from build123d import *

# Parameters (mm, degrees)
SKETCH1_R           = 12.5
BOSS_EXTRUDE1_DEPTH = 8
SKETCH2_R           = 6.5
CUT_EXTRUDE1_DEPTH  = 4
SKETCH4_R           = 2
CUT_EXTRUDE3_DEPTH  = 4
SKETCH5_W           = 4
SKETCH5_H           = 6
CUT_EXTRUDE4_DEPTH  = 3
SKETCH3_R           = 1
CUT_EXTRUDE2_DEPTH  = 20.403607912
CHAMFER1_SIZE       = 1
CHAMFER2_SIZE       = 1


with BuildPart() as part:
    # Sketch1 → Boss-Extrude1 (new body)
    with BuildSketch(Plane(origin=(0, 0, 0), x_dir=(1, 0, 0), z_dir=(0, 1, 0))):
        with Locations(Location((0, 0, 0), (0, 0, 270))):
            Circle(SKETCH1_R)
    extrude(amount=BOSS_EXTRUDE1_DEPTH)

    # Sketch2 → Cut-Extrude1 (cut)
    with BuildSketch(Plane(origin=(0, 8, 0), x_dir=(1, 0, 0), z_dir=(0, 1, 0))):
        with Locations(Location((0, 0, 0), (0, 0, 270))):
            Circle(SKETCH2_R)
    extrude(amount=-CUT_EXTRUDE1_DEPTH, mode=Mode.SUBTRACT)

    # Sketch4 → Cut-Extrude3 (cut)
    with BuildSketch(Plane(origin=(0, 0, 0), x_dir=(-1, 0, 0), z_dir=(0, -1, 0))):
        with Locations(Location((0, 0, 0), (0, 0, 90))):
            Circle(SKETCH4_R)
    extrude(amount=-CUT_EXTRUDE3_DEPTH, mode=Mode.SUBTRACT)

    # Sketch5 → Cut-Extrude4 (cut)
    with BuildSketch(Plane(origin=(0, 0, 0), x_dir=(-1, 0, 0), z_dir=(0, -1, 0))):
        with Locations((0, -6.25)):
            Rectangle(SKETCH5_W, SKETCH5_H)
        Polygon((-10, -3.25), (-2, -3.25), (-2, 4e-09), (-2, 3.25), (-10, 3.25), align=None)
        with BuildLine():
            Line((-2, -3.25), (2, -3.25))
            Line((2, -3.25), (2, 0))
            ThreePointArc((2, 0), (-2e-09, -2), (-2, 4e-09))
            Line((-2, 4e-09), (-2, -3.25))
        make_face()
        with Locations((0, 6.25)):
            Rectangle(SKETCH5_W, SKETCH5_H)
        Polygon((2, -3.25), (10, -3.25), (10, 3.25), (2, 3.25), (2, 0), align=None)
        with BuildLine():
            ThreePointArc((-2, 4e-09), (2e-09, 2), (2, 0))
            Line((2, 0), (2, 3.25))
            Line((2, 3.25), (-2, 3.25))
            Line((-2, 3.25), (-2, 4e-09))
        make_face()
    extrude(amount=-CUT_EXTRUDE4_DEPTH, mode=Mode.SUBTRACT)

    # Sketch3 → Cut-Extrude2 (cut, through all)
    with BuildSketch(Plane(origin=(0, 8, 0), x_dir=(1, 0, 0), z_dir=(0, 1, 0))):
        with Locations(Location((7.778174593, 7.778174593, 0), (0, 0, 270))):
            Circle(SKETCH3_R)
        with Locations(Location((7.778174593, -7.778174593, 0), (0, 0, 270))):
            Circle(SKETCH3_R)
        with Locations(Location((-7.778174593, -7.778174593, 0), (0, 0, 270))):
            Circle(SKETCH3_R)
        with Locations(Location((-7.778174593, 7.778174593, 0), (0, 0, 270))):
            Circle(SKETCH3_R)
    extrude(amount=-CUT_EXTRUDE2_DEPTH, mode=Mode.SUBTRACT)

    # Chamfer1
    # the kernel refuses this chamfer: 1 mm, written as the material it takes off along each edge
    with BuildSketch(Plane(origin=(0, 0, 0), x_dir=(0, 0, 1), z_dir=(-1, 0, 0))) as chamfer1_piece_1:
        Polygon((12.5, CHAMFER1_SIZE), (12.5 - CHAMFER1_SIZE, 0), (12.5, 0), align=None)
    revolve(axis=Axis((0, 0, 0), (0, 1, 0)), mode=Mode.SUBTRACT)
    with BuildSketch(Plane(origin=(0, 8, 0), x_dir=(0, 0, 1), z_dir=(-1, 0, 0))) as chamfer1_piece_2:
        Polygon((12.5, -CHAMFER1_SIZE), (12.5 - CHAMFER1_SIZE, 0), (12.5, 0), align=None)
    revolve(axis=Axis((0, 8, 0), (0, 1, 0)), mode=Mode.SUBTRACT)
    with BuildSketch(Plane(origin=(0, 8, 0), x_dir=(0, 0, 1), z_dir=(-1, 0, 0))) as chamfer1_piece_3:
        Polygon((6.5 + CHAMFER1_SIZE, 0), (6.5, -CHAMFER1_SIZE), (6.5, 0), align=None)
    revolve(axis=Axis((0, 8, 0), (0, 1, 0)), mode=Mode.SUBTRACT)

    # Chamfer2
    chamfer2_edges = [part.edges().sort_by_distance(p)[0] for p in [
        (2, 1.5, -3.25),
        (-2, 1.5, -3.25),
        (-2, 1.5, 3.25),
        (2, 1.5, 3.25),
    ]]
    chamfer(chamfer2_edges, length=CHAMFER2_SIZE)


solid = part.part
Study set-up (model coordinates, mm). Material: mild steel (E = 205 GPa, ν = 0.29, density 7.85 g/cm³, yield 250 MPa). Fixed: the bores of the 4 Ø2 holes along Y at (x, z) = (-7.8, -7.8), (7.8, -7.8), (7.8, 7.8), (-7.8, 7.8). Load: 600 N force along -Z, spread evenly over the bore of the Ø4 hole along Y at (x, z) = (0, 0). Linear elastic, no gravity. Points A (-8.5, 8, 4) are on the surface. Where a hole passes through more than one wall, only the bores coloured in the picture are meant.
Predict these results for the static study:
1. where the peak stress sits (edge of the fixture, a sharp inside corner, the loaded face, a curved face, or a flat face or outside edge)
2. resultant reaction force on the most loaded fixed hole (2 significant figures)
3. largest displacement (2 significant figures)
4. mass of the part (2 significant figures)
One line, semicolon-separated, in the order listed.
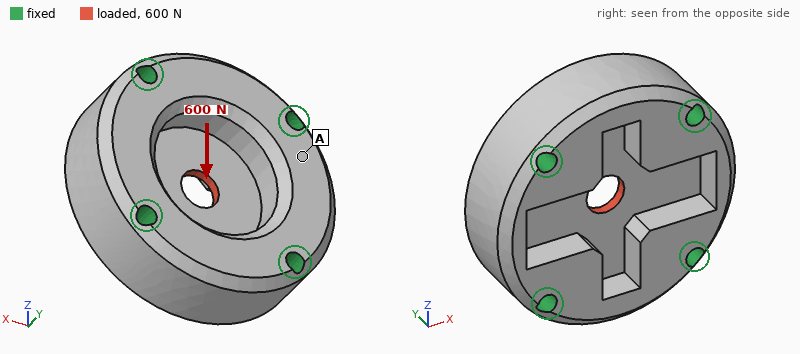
the loaded face; 150 N; 1.1 µm; 21 g
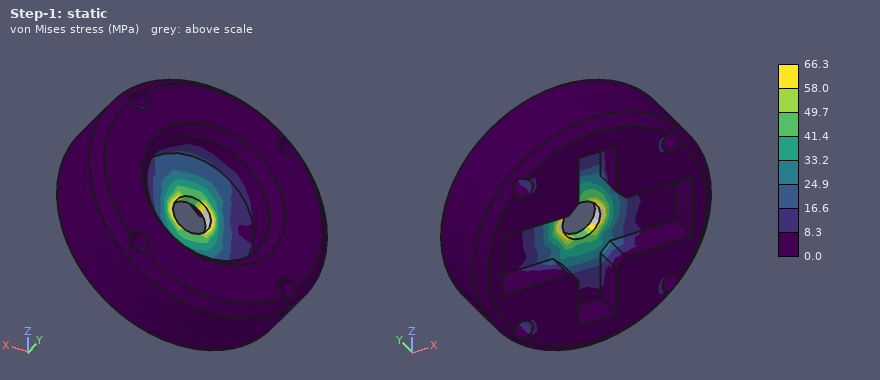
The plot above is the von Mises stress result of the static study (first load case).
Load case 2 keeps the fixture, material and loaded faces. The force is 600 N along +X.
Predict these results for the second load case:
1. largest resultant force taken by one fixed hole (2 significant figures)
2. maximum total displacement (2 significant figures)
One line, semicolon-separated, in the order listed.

160 N; 1.1 µm
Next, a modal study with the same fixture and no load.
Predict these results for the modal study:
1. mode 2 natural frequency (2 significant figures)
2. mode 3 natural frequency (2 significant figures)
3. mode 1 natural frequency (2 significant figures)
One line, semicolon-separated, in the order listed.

73 kHz; 75 kHz; 72 kHz
